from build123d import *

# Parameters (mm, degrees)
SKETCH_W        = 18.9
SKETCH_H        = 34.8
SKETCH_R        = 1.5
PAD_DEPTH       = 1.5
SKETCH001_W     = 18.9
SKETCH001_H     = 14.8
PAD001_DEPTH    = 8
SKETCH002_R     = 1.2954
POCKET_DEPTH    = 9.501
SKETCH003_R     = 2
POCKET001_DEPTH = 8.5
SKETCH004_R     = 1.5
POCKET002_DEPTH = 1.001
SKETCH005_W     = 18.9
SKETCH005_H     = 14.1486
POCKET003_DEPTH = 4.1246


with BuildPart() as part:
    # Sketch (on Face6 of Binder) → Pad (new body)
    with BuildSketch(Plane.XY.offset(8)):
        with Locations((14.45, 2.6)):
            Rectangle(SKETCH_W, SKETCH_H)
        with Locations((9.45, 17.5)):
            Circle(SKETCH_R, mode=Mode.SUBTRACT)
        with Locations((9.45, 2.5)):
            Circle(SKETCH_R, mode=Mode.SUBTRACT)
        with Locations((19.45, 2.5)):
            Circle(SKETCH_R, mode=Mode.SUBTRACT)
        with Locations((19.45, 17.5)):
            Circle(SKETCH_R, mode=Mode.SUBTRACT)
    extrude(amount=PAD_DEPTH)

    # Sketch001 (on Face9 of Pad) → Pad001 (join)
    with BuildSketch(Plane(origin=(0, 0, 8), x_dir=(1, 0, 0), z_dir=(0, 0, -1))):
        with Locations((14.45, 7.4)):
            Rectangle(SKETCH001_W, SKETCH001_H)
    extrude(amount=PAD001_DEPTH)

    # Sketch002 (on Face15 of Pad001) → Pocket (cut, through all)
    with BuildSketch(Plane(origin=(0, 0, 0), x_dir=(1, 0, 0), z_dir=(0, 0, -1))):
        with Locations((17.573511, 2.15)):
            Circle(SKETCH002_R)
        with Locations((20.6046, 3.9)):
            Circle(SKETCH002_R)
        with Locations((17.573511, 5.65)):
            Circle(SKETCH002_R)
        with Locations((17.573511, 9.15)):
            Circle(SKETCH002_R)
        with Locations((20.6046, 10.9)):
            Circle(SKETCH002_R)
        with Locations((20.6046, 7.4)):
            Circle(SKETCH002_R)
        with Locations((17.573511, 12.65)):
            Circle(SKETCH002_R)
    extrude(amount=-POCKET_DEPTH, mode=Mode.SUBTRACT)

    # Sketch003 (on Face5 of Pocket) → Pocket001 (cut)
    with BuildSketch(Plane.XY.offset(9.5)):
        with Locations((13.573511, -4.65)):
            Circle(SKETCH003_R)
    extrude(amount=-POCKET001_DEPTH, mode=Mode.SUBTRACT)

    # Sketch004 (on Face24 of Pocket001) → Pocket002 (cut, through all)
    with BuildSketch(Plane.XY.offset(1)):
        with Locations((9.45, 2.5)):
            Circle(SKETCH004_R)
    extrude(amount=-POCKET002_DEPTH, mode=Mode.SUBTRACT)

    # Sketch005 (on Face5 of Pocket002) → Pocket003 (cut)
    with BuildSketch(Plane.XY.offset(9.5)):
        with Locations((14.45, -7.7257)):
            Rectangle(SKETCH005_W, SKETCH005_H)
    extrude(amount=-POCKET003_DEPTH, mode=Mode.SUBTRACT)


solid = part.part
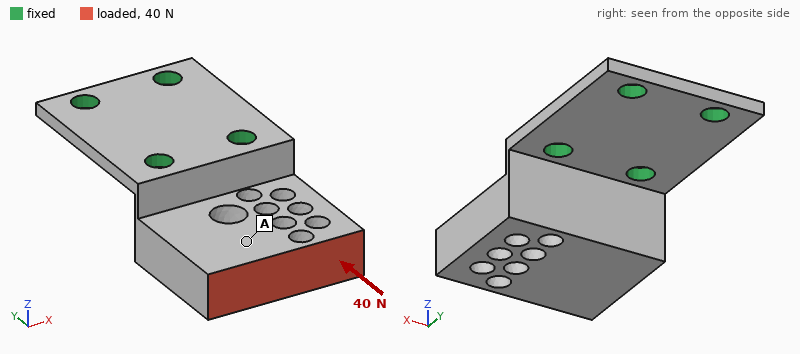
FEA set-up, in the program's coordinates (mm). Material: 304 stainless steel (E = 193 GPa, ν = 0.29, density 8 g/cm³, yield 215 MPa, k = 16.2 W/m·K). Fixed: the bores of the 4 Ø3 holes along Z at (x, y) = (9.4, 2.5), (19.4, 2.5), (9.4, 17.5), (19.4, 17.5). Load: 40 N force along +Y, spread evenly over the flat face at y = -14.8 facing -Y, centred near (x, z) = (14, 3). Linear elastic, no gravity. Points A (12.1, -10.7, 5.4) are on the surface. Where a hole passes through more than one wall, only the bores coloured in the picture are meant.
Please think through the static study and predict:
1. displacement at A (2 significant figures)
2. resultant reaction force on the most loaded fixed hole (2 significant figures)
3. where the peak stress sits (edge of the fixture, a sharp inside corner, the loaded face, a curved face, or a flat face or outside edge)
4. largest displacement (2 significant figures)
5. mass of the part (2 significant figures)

62 µm
19 N
a flat face or outside edge
95 µm
15 g
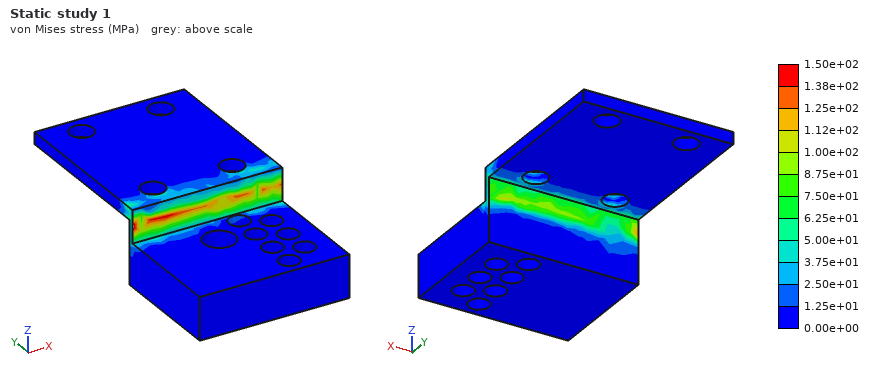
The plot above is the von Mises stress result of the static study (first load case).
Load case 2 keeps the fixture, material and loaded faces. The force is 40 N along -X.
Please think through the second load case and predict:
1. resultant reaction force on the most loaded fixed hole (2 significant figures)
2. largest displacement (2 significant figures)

53 N
13 µm
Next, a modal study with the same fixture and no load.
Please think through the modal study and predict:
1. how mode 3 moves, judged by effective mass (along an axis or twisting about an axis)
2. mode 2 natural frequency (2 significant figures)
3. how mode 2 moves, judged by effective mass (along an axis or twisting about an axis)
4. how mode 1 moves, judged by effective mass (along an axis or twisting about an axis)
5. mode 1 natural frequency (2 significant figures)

along Y
4500 Hz
along X
along Z
870 Hz
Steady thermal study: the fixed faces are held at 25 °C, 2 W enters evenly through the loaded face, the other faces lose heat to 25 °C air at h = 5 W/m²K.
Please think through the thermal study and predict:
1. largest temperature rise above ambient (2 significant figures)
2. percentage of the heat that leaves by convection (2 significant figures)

66 K
15 %
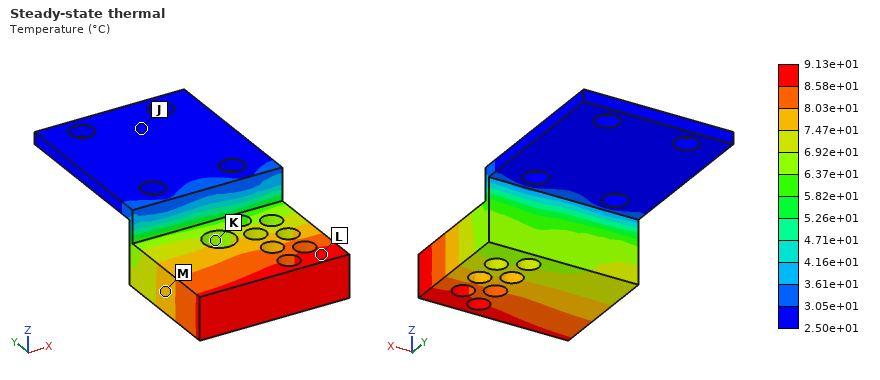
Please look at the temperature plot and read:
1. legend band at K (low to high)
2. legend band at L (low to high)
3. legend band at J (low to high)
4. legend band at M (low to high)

6.37e+01 to 6.92e+01 °C
8.58e+01 to 9.13e+01 °C
2.50e+01 to 3.05e+01 °C
7.47e+01 to 8.03e+01 °C
